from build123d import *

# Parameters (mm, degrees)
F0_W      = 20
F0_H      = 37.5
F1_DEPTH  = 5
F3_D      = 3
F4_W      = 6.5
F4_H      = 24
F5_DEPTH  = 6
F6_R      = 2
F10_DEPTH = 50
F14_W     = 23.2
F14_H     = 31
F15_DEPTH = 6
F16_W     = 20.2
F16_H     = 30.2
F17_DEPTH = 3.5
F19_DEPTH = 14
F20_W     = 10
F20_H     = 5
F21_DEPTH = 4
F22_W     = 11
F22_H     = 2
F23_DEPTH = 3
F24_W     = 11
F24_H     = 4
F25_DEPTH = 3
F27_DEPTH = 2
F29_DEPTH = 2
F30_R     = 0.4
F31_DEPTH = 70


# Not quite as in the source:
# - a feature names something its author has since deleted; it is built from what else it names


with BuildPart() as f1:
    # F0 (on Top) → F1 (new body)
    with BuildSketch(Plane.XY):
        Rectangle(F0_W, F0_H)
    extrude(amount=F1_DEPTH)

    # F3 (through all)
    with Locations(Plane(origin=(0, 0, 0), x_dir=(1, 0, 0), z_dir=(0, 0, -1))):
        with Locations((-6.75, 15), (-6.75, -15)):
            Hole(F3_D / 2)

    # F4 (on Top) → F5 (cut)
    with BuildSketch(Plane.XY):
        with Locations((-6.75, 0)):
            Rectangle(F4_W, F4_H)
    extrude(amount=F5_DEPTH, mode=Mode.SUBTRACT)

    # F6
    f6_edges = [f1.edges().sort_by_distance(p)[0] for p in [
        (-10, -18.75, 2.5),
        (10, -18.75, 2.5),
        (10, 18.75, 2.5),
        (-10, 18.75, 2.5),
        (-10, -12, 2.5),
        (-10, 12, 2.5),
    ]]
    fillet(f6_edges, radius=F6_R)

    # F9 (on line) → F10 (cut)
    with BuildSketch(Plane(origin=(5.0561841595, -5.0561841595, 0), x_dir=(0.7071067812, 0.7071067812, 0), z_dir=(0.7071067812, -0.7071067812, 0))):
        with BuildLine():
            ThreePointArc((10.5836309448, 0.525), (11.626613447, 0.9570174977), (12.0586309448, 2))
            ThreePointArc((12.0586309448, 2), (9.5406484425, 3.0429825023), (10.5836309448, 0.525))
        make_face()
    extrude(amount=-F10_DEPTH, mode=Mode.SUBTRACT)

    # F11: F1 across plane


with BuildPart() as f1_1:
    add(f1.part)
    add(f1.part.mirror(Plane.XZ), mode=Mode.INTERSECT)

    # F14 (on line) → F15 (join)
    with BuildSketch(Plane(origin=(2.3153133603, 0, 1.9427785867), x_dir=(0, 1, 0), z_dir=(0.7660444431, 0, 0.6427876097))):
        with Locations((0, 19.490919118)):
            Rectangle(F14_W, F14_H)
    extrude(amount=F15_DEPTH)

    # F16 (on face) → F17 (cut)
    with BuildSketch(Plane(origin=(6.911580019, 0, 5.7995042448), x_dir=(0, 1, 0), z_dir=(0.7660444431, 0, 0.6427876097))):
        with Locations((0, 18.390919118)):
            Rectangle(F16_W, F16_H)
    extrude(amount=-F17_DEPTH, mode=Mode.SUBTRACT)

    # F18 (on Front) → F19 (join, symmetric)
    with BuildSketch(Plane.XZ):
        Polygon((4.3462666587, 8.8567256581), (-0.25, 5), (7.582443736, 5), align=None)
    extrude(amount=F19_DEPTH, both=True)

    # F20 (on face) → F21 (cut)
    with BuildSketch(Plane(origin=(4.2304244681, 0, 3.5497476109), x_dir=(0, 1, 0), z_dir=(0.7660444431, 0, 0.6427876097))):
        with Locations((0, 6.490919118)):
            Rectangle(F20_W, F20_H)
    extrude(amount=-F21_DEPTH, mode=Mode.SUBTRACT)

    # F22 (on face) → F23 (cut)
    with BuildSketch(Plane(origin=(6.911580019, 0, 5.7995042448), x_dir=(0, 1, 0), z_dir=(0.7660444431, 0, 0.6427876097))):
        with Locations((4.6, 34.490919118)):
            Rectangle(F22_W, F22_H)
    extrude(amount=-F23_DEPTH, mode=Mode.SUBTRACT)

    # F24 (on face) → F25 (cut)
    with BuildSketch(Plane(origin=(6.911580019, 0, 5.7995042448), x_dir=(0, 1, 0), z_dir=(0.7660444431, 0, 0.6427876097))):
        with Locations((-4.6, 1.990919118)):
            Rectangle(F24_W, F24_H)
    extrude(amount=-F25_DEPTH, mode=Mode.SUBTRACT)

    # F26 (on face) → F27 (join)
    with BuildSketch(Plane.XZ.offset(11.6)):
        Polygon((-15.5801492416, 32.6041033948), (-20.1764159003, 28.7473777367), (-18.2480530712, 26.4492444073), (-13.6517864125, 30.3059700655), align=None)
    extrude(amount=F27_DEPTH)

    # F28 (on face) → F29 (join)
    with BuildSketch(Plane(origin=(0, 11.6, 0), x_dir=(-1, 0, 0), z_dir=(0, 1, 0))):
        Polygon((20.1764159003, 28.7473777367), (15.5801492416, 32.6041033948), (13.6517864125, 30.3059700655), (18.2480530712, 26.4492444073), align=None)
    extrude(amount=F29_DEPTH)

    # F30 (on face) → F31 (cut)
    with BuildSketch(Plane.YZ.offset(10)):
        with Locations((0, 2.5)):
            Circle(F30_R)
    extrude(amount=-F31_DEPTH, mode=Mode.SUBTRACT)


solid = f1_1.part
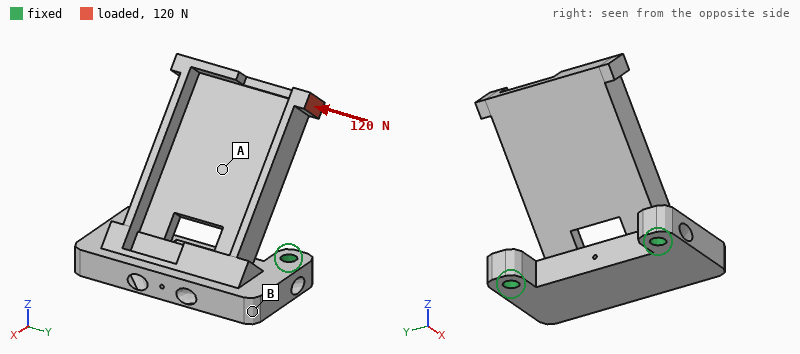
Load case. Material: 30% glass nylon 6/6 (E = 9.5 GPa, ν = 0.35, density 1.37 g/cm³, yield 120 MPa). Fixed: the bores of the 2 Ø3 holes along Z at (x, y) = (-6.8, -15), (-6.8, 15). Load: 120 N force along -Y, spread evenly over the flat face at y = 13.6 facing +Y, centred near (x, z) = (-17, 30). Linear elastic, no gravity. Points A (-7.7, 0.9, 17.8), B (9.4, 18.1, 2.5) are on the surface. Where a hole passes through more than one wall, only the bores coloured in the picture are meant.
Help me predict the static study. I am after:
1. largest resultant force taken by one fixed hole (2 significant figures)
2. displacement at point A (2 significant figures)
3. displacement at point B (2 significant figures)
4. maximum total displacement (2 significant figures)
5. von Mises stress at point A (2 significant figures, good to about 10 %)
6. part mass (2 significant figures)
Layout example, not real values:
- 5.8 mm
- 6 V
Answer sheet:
- 140 N
- 0.077 mm
- 0.050 mm
- 0.32 mm
- 12 MPa
- 6.9 g
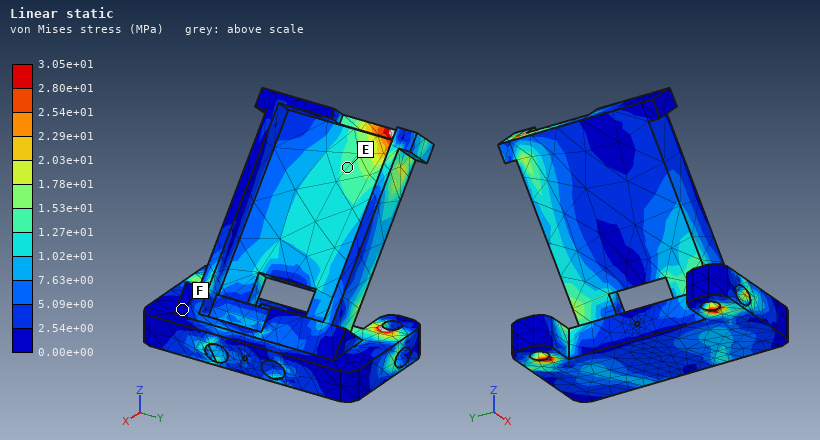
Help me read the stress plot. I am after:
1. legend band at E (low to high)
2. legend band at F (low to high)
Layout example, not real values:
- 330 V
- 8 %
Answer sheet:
- 1.27e+01 to 1.53e+01 MPa
- 0.00e+00 to 2.54e+00 MPa
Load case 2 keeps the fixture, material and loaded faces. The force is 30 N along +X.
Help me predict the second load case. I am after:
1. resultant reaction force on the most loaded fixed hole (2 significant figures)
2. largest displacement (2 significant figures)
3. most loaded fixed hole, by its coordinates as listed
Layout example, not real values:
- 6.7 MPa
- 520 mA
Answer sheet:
- 29 N
- 0.64 mm
- (-6.8, 15)
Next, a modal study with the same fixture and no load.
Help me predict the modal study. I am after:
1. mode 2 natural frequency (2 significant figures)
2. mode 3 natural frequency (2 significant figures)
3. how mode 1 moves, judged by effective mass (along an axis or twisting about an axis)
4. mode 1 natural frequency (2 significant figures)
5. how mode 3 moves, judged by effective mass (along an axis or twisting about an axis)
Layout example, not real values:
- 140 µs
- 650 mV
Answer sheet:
- 2800 Hz
- 3700 Hz
- along X
- 1100 Hz
- along Y
